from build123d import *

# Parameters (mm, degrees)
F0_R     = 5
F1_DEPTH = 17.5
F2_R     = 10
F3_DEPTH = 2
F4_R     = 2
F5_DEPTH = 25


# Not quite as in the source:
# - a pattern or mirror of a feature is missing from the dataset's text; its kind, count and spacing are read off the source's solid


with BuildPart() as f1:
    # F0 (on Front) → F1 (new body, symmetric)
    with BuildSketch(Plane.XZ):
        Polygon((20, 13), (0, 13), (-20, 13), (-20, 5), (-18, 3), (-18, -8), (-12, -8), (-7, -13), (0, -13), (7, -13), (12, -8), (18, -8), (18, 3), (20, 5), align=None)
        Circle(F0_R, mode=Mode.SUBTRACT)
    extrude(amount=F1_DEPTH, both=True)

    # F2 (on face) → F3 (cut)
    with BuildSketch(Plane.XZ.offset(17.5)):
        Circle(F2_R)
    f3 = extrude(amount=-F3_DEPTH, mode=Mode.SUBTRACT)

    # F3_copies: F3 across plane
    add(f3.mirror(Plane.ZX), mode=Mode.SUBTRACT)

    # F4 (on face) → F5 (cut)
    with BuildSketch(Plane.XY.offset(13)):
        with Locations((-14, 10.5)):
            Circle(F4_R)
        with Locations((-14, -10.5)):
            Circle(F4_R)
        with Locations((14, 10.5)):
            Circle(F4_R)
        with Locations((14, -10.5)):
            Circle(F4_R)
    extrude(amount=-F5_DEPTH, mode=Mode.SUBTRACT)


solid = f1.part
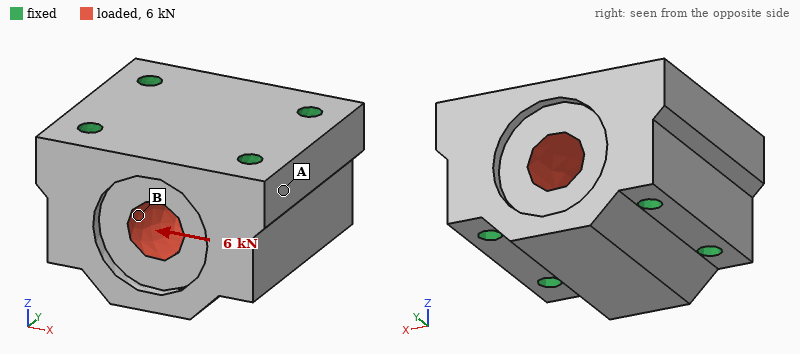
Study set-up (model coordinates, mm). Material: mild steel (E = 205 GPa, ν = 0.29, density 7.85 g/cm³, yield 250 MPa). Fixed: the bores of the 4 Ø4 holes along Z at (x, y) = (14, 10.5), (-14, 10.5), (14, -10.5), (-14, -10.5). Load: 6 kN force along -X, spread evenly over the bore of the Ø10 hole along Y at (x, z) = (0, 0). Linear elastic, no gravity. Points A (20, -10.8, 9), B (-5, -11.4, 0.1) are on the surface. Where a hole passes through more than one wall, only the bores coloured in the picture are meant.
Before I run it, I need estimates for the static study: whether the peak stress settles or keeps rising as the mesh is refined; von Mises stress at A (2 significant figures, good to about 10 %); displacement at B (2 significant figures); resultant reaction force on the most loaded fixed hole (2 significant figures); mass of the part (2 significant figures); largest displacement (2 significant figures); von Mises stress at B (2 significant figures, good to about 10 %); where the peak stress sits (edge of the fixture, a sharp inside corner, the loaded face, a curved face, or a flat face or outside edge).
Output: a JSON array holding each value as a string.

["keeps rising", "2.4 MPa", "0.27 µm", "1.5 kN", "210 g", "0.51 µm", "6.7 MPa", "edge of the fixture"]
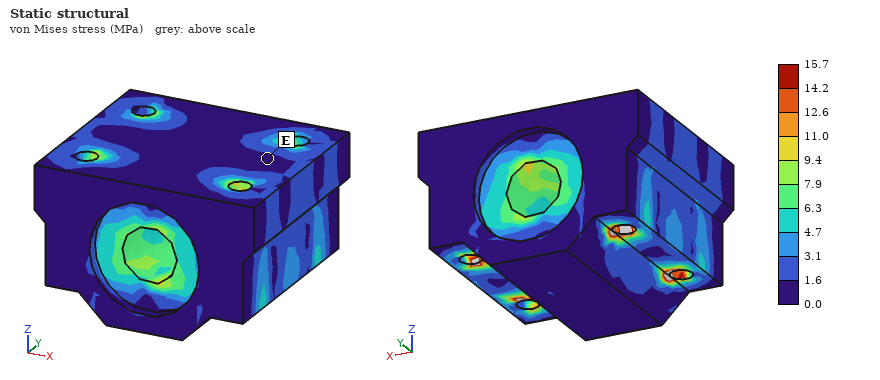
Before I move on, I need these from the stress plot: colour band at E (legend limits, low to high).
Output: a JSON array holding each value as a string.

["0.0 to 1.6 MPa"]
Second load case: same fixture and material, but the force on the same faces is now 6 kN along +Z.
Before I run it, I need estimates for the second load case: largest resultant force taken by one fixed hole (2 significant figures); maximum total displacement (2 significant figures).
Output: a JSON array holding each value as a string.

["1.5 kN", "0.90 µm"]
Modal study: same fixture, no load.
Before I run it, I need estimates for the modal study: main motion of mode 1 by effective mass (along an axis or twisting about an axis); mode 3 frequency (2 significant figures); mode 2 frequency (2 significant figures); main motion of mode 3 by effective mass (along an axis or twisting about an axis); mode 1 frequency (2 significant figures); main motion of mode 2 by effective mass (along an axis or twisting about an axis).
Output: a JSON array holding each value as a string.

["along Y", "54 kHz", "48 kHz", "along Y", "45 kHz", "along Z"]
